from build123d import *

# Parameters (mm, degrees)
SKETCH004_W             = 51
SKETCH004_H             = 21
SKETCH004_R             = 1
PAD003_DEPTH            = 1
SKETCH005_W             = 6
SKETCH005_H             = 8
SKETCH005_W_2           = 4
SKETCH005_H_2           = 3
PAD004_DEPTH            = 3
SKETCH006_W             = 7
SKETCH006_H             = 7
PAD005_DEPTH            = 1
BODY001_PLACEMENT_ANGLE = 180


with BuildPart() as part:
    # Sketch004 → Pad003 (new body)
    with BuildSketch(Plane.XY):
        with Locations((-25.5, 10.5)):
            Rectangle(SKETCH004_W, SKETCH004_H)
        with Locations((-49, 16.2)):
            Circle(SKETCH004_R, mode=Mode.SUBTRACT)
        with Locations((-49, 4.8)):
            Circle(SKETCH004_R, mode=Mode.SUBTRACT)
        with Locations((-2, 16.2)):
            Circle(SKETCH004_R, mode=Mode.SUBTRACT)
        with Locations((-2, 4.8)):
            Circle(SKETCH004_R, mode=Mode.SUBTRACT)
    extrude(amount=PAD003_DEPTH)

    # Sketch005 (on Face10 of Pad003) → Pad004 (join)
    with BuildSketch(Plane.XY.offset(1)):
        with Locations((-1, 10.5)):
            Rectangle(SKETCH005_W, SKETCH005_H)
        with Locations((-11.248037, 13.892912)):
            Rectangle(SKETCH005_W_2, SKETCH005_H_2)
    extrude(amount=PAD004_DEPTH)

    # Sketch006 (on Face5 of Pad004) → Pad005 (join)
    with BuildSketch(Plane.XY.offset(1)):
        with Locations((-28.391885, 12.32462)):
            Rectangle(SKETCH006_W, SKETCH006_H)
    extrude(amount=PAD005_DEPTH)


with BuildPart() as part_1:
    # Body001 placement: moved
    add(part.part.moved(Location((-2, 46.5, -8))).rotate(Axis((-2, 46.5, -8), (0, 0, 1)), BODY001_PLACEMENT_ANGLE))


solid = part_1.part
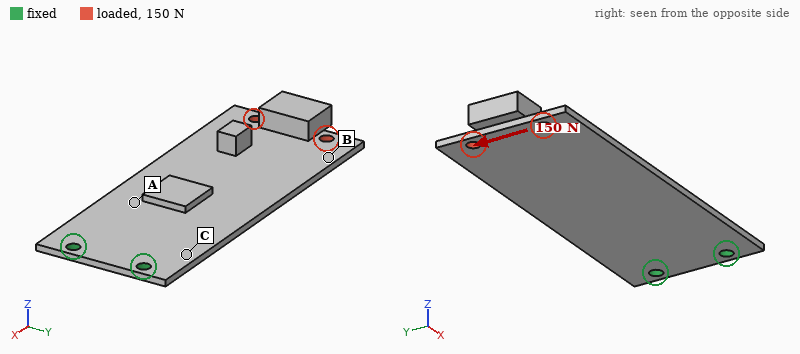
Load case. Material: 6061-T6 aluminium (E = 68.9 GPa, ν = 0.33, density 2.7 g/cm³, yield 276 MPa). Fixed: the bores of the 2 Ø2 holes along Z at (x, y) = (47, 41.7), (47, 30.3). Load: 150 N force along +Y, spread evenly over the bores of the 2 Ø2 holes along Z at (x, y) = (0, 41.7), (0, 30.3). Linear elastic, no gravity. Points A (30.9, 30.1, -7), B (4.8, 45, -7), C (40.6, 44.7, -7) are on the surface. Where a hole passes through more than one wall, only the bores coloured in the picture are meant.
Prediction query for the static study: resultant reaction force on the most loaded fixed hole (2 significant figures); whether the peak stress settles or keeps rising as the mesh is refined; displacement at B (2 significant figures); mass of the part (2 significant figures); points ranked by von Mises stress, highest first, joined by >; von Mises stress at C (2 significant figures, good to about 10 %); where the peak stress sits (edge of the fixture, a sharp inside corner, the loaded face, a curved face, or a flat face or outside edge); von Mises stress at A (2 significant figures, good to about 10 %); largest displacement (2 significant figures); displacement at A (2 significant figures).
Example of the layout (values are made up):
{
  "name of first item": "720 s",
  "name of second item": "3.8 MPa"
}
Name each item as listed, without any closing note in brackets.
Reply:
{
  "resultant reaction force on the most loaded fixed hole": "560 N",
  "whether the peak stress settles or keeps rising as the mesh is refined": "keeps rising",
  "displacement at B": "0.13 mm",
  "mass of the part": "3.5 g",
  "points ranked by von Mises stress, highest first, joined by >": "C > A > B",
  "von Mises stress at C": "64 MPa",
  "where the peak stress sits": "edge of the fixture",
  "von Mises stress at A": "42 MPa",
  "largest displacement": "0.16 mm",
  "displacement at A": "0.034 mm"
}
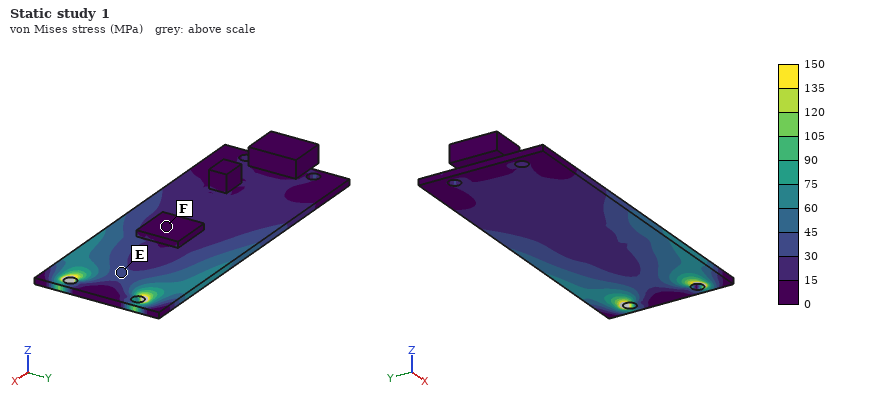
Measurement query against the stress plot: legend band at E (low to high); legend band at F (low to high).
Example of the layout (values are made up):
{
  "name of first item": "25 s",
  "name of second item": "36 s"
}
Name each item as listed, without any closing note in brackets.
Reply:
{
  "legend band at E": "30 to 45 MPa",
  "legend band at F": "0 to 15 MPa"
}
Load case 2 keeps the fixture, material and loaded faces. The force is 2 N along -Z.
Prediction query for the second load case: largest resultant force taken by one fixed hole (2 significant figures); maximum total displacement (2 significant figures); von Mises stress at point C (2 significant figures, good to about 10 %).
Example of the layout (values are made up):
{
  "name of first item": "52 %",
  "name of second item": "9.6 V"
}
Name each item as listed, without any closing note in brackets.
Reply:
{
  "largest resultant force taken by one fixed hole": "1.1 N",
  "maximum total displacement": "0.58 mm",
  "von Mises stress at point C": "23 MPa"
}
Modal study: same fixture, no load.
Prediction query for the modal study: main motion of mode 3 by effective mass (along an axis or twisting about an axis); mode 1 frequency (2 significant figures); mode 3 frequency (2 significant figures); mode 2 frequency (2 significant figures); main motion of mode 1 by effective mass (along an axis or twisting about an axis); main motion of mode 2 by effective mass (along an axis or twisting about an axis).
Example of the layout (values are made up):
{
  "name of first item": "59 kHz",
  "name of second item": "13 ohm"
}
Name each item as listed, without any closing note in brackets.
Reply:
{
  "main motion of mode 3 by effective mass": "along Z",
  "mode 1 frequency": "280 Hz",
  "mode 3 frequency": "1900 Hz",
  "mode 2 frequency": "1800 Hz",
  "main motion of mode 1 by effective mass": "along Z",
  "main motion of mode 2 by effective mass": "twisting about X"
}
